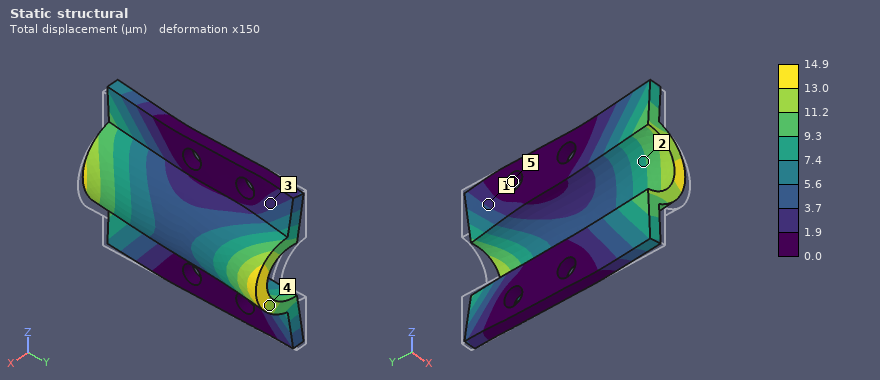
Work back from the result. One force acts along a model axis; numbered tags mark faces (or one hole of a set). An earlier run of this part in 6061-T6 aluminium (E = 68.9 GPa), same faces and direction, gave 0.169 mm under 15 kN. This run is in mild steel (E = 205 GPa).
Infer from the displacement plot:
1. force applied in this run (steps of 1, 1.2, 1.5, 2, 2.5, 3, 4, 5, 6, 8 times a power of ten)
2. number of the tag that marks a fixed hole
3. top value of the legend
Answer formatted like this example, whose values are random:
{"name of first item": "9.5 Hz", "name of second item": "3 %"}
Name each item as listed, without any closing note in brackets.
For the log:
{"force applied in this run": "4 kN", "number of the tag that marks a fixed hole": "5", "top value of the legend": "14.9 µm"}
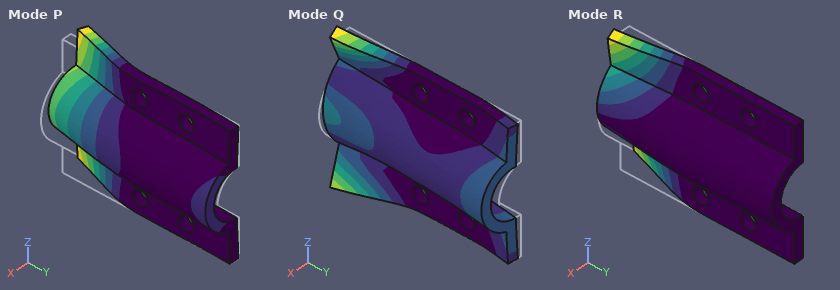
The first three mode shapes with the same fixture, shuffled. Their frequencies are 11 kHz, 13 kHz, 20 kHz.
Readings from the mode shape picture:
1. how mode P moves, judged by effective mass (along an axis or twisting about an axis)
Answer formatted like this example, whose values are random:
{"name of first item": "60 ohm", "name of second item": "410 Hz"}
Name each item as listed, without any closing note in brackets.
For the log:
{"how mode P moves, judged by effective mass": "along X"}
